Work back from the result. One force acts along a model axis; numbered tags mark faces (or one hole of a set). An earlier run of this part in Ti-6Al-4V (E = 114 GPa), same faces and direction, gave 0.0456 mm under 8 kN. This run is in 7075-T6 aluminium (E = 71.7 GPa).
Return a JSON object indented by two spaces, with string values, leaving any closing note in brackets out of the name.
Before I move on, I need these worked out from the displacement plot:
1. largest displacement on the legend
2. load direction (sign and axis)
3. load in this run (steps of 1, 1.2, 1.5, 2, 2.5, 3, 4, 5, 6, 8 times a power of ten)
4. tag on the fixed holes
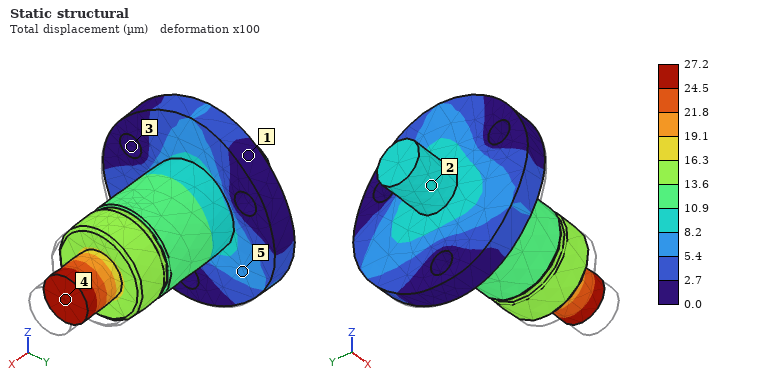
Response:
{
  "largest displacement on the legend": "27.2 µm",
  "load direction": "-X",
  "load in this run": "3 kN",
  "tag on the fixed holes": "3"
}
